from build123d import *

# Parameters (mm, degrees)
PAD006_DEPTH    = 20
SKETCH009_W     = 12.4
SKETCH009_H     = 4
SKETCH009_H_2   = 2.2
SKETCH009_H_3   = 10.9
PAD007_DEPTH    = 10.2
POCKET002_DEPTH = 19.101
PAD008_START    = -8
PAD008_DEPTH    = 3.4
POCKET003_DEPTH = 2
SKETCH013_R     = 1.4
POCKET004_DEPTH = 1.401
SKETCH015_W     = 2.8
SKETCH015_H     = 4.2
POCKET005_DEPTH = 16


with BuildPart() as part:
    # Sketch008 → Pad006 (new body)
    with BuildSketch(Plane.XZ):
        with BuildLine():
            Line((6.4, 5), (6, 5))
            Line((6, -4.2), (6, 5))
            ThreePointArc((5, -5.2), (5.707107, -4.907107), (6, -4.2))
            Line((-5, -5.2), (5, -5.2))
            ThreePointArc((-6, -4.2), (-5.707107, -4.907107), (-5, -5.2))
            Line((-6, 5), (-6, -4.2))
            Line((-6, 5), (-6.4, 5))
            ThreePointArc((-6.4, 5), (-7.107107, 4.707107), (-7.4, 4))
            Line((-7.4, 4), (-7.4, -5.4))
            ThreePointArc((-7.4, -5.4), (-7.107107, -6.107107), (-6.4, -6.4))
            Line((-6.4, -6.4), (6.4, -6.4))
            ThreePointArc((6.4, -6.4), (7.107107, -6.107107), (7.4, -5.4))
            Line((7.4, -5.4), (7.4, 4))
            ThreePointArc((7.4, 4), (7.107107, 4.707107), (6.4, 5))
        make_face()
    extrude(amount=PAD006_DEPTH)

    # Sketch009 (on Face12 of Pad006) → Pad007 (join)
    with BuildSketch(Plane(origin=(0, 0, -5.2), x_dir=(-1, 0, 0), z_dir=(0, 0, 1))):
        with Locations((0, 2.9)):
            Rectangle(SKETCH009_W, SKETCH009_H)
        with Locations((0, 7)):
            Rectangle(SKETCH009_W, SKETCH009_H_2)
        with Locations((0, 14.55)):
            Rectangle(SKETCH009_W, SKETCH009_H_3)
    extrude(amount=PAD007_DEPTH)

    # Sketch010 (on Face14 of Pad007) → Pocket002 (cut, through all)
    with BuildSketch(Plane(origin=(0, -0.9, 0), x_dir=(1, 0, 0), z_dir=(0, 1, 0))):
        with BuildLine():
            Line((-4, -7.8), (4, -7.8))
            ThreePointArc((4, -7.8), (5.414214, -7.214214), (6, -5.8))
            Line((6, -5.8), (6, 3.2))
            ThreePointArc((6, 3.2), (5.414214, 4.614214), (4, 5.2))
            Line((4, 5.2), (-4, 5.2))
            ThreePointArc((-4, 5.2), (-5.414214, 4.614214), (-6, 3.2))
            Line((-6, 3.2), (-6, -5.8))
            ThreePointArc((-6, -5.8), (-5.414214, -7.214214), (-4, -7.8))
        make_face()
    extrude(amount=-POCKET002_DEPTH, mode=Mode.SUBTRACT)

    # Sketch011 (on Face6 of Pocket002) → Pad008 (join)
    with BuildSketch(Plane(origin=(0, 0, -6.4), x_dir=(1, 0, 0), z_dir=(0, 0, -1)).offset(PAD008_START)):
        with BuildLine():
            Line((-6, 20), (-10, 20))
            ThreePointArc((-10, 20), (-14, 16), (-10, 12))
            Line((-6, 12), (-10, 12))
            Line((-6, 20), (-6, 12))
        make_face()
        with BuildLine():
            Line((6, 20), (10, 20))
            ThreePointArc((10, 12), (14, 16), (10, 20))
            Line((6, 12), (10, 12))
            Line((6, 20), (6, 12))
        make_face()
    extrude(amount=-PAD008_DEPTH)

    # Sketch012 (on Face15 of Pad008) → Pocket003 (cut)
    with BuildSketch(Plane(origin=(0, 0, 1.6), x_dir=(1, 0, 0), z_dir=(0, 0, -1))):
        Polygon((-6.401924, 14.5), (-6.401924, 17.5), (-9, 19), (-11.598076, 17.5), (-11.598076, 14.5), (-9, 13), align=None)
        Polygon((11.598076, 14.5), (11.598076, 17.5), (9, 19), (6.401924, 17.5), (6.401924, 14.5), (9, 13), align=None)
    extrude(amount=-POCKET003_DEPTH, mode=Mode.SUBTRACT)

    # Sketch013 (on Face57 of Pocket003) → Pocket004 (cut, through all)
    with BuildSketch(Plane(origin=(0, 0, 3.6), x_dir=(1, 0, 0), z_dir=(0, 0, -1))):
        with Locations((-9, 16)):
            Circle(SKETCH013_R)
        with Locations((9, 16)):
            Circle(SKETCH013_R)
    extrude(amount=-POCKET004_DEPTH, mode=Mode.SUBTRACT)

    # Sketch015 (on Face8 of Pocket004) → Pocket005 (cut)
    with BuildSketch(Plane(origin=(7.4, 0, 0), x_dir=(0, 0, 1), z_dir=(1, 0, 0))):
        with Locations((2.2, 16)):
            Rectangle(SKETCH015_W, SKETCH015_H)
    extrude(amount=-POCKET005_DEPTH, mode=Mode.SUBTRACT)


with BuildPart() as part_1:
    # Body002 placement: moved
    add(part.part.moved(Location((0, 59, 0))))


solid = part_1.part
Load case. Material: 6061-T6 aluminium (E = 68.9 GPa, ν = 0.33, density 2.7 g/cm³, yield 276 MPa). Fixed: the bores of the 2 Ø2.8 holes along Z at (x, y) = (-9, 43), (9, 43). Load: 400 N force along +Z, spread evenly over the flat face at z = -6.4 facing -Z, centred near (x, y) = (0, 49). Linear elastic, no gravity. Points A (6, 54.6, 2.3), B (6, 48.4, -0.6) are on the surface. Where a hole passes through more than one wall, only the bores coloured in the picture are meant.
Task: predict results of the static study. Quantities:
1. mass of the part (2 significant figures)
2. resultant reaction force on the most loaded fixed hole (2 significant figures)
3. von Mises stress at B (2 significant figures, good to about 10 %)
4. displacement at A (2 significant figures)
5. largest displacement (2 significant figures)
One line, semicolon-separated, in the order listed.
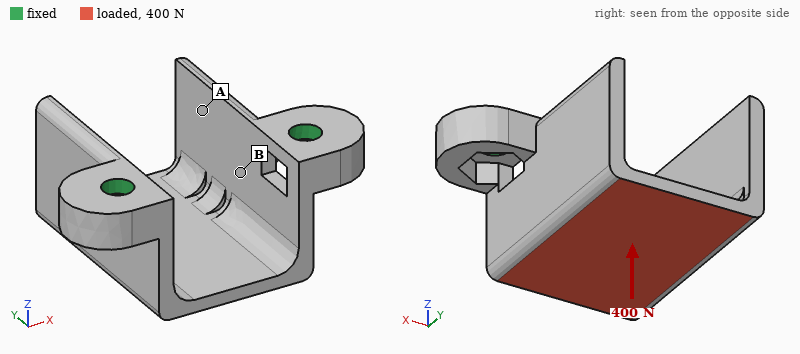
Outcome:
3.0 g; 210 N; 47 MPa; 0.069 mm; 0.13 mm
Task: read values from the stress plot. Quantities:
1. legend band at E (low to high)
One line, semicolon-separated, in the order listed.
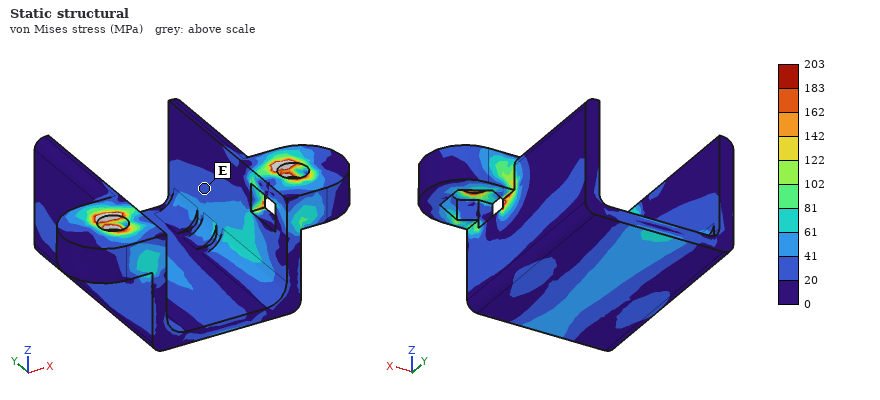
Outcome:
20 to 41 MPa
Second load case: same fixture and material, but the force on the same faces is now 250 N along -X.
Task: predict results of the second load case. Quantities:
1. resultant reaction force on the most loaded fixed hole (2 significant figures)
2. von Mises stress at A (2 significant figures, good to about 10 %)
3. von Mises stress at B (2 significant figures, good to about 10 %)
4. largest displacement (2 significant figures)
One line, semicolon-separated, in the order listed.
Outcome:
180 N; 13 MPa; 36 MPa; 73 µm
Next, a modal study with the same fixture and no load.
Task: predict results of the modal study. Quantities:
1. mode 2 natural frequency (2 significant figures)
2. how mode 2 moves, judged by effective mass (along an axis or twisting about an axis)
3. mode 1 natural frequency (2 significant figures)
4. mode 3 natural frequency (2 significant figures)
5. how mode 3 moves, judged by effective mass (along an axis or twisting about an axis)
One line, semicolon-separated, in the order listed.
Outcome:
6500 Hz; along X; 5800 Hz; 9900 Hz; along X
